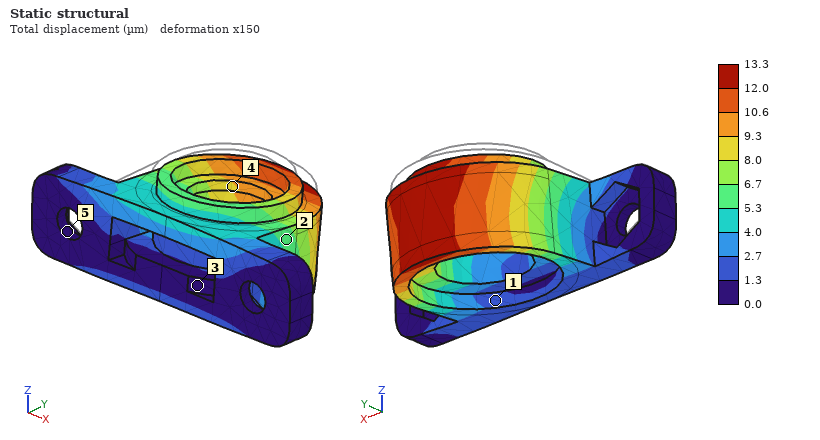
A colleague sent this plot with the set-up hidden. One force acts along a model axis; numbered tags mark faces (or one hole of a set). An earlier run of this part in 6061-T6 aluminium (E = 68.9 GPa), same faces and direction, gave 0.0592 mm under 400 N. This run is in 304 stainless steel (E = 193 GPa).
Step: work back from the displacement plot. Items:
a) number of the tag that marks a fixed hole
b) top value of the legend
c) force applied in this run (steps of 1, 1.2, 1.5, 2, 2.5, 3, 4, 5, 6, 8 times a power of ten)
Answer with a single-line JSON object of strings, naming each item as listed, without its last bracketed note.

{"number of the tag that marks a fixed hole": "5", "top value of the legend": "13.3 µm", "force applied in this run": "250 N"}
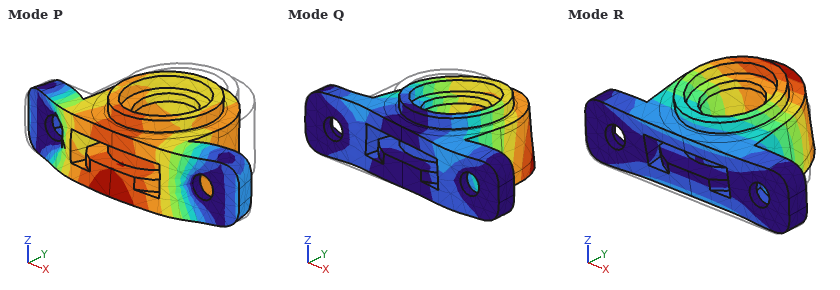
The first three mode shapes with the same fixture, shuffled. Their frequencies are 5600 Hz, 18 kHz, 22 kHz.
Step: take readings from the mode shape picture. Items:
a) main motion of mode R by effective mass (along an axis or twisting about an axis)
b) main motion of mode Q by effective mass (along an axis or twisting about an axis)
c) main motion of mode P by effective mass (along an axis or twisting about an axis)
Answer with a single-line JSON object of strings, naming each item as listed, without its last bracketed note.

{"main motion of mode R by effective mass": "along Z", "main motion of mode Q by effective mass": "along X", "main motion of mode P by effective mass": "along Y"}
